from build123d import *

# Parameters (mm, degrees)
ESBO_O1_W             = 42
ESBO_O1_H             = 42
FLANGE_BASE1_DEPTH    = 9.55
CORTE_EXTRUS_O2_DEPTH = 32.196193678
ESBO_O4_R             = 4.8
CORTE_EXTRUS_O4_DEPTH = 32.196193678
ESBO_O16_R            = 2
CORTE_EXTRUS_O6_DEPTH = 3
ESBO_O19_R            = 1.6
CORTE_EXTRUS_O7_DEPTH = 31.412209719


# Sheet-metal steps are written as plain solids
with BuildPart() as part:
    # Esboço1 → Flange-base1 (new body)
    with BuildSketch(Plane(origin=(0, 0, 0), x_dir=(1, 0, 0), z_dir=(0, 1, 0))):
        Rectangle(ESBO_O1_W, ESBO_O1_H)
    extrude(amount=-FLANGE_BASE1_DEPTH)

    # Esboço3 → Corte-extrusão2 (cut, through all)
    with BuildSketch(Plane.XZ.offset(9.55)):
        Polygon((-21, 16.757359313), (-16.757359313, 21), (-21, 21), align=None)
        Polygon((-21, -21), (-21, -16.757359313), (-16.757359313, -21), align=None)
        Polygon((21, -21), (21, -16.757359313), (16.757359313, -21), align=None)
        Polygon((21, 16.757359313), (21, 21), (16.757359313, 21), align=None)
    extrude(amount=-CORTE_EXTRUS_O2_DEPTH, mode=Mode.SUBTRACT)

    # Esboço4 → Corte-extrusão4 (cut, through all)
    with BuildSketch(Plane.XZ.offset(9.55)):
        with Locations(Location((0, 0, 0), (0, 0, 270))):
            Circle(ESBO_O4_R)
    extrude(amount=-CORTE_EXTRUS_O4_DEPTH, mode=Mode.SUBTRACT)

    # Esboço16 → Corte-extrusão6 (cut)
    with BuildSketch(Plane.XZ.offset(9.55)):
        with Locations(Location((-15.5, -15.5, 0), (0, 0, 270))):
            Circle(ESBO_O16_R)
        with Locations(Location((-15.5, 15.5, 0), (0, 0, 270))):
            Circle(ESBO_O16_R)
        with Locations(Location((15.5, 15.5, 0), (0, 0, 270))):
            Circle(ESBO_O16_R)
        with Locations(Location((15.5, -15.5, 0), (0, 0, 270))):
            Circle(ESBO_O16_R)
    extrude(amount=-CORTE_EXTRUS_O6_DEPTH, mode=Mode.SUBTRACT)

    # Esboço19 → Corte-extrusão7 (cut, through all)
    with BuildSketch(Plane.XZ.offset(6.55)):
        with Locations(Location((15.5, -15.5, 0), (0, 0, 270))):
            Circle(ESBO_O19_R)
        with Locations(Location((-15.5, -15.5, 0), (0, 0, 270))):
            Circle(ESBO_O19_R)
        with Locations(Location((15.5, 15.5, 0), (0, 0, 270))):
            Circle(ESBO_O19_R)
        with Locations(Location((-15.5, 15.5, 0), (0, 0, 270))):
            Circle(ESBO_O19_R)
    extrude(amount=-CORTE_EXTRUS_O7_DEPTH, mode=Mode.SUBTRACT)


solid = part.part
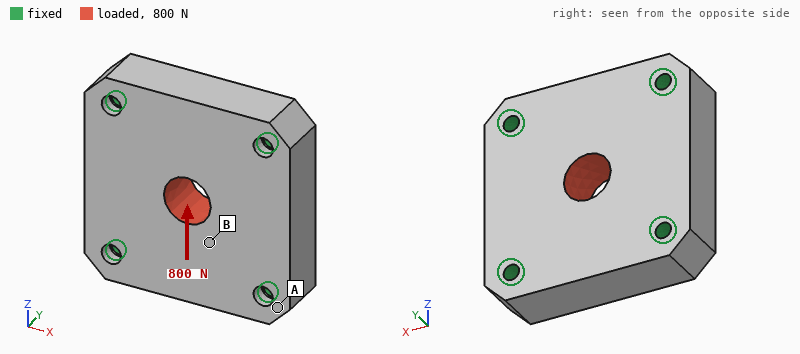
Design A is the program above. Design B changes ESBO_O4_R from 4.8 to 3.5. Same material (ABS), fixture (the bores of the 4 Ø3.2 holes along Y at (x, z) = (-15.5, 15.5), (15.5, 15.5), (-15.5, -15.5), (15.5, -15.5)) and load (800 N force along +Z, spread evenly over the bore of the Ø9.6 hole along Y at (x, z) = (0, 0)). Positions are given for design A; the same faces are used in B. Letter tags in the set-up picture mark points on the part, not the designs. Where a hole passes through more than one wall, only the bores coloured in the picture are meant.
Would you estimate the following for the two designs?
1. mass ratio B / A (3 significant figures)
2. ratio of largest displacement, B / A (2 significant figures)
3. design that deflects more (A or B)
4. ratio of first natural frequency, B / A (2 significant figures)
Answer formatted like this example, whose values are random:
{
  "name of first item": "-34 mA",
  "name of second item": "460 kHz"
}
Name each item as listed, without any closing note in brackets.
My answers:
{
  "mass ratio B / A": "1.02",
  "ratio of largest displacement, B / A": "1.1",
  "design that deflects more": "B",
  "ratio of first natural frequency, B / A": "0.99"
}
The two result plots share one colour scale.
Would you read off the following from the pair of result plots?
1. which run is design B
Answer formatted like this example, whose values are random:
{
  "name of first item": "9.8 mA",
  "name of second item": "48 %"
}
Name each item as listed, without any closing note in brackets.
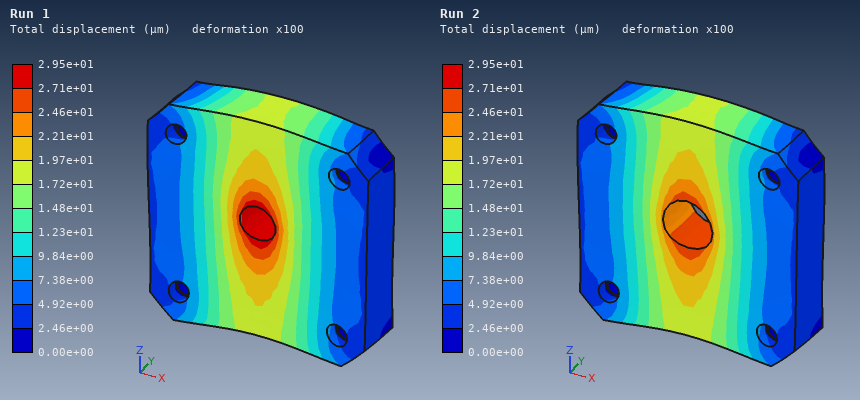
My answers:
{
  "which run is design B": "Run 1"
}
